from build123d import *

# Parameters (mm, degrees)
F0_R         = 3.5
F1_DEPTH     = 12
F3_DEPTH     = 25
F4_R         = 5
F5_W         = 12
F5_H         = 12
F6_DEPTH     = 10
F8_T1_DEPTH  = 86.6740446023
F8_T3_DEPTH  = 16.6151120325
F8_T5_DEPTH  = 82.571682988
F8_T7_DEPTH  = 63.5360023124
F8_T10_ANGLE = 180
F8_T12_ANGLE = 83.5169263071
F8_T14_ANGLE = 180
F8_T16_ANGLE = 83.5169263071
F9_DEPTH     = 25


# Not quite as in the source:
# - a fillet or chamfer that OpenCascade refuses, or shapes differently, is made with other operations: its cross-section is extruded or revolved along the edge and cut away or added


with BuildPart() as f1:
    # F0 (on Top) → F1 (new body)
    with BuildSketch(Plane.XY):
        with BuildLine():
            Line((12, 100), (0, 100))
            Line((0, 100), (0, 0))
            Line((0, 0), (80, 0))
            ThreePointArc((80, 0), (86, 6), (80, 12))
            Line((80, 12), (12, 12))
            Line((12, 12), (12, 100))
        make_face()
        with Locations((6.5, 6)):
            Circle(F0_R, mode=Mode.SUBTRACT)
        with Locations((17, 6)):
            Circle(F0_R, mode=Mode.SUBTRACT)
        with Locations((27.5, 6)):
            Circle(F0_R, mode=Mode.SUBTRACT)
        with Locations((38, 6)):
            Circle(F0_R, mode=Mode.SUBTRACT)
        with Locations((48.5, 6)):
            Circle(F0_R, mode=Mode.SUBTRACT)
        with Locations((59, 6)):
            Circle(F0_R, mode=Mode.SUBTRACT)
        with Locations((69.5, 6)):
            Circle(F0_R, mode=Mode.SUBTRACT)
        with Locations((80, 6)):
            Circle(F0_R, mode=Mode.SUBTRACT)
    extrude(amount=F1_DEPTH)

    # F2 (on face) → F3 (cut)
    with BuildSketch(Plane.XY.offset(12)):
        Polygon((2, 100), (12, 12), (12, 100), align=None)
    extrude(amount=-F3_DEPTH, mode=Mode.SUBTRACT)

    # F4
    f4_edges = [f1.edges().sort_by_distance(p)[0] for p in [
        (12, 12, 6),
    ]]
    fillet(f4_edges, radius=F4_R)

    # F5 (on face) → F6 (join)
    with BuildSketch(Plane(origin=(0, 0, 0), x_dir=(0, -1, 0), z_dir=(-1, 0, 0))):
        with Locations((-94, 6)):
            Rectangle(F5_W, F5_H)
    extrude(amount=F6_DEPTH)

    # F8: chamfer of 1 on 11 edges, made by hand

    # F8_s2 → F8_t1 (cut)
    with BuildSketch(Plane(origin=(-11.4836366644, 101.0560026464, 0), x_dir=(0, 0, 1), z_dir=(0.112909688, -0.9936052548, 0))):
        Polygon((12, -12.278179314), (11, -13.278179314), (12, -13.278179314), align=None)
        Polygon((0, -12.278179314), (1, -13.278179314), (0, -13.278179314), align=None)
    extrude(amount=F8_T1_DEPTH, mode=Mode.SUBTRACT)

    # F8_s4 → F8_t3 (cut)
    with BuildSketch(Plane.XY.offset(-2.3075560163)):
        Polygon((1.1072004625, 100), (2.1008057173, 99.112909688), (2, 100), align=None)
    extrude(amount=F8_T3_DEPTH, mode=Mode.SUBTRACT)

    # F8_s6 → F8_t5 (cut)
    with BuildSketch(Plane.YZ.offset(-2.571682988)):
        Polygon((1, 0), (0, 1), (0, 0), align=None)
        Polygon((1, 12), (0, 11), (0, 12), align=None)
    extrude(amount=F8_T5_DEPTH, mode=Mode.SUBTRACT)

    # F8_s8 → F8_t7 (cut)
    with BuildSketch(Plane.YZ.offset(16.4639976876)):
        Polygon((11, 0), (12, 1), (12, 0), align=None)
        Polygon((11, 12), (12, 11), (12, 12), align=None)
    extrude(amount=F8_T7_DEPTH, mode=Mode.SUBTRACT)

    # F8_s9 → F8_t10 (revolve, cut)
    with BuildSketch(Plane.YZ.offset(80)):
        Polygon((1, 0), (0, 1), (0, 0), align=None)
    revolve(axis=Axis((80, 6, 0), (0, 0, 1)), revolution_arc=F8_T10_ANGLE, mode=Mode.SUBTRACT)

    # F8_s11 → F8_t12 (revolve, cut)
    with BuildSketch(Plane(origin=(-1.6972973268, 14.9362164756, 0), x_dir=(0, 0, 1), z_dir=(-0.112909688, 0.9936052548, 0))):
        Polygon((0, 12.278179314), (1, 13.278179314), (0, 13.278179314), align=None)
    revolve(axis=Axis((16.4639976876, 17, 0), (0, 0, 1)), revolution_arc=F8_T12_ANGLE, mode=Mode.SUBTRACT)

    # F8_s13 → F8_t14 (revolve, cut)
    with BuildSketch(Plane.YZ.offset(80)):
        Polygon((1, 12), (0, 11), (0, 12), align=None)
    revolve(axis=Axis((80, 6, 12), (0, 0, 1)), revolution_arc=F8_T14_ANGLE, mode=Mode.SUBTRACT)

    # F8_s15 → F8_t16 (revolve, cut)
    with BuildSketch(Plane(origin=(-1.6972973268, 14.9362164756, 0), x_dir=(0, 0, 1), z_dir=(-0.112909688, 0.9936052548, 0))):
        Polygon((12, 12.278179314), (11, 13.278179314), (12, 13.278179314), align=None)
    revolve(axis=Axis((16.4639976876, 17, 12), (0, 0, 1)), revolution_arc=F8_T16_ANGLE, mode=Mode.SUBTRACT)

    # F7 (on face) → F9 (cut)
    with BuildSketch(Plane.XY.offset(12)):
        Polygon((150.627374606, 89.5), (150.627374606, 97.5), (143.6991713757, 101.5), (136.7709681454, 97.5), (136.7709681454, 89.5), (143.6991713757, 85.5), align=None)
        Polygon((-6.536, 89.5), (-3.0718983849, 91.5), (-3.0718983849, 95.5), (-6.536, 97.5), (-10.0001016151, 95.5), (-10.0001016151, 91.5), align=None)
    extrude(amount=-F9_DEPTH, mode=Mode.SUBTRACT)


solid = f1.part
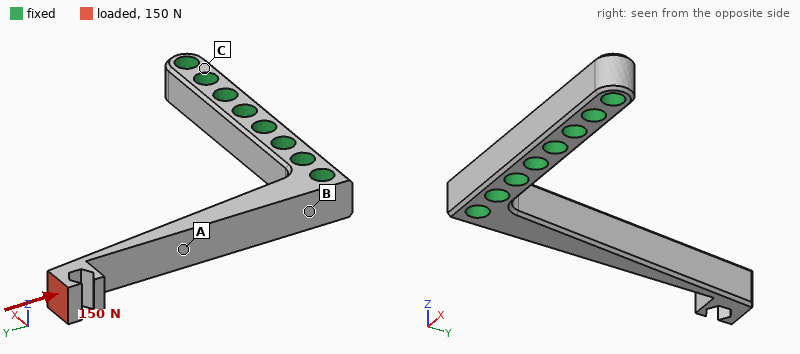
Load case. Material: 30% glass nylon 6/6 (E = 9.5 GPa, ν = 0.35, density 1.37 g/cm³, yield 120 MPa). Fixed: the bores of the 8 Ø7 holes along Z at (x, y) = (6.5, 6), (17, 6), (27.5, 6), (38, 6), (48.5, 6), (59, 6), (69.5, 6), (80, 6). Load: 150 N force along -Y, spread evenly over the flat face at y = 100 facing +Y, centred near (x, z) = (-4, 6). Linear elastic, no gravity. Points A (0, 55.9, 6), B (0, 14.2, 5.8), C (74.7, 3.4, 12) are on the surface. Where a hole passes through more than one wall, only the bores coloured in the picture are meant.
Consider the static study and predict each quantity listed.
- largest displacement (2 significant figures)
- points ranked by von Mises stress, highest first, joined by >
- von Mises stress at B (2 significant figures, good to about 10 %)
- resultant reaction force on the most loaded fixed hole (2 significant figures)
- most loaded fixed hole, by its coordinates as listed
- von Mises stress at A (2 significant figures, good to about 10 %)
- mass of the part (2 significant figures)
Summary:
1.5 mm
A > B > C
6.0 MPa
240 N
(6.5, 6)
14 MPa
23 g
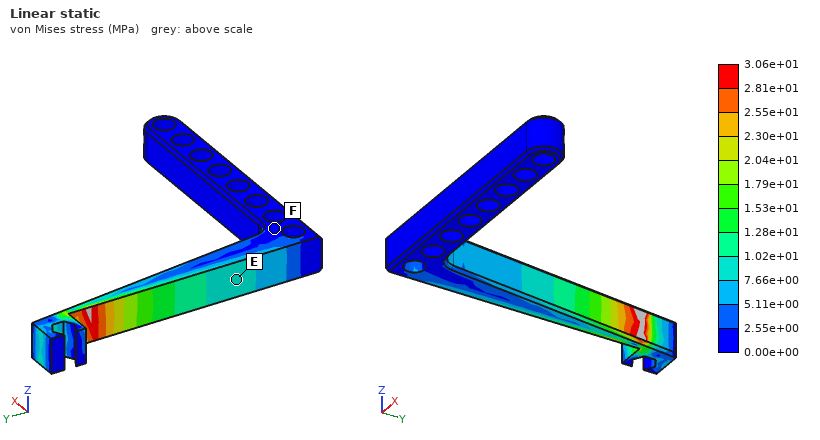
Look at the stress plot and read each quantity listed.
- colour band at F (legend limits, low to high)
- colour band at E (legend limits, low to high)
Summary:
0.00e+00 to 2.55e+00 MPa
7.66e+00 to 1.02e+01 MPa
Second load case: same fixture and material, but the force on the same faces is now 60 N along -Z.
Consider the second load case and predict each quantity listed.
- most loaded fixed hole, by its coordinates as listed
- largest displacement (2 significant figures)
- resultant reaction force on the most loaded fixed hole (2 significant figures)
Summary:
(6.5, 6)
1.4 mm
68 N
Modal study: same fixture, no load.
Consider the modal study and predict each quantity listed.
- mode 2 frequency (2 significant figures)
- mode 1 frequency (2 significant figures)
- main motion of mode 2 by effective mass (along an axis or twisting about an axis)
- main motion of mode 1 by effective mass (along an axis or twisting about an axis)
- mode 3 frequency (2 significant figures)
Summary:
720 Hz
550 Hz
along Z
along X
2000 Hz
